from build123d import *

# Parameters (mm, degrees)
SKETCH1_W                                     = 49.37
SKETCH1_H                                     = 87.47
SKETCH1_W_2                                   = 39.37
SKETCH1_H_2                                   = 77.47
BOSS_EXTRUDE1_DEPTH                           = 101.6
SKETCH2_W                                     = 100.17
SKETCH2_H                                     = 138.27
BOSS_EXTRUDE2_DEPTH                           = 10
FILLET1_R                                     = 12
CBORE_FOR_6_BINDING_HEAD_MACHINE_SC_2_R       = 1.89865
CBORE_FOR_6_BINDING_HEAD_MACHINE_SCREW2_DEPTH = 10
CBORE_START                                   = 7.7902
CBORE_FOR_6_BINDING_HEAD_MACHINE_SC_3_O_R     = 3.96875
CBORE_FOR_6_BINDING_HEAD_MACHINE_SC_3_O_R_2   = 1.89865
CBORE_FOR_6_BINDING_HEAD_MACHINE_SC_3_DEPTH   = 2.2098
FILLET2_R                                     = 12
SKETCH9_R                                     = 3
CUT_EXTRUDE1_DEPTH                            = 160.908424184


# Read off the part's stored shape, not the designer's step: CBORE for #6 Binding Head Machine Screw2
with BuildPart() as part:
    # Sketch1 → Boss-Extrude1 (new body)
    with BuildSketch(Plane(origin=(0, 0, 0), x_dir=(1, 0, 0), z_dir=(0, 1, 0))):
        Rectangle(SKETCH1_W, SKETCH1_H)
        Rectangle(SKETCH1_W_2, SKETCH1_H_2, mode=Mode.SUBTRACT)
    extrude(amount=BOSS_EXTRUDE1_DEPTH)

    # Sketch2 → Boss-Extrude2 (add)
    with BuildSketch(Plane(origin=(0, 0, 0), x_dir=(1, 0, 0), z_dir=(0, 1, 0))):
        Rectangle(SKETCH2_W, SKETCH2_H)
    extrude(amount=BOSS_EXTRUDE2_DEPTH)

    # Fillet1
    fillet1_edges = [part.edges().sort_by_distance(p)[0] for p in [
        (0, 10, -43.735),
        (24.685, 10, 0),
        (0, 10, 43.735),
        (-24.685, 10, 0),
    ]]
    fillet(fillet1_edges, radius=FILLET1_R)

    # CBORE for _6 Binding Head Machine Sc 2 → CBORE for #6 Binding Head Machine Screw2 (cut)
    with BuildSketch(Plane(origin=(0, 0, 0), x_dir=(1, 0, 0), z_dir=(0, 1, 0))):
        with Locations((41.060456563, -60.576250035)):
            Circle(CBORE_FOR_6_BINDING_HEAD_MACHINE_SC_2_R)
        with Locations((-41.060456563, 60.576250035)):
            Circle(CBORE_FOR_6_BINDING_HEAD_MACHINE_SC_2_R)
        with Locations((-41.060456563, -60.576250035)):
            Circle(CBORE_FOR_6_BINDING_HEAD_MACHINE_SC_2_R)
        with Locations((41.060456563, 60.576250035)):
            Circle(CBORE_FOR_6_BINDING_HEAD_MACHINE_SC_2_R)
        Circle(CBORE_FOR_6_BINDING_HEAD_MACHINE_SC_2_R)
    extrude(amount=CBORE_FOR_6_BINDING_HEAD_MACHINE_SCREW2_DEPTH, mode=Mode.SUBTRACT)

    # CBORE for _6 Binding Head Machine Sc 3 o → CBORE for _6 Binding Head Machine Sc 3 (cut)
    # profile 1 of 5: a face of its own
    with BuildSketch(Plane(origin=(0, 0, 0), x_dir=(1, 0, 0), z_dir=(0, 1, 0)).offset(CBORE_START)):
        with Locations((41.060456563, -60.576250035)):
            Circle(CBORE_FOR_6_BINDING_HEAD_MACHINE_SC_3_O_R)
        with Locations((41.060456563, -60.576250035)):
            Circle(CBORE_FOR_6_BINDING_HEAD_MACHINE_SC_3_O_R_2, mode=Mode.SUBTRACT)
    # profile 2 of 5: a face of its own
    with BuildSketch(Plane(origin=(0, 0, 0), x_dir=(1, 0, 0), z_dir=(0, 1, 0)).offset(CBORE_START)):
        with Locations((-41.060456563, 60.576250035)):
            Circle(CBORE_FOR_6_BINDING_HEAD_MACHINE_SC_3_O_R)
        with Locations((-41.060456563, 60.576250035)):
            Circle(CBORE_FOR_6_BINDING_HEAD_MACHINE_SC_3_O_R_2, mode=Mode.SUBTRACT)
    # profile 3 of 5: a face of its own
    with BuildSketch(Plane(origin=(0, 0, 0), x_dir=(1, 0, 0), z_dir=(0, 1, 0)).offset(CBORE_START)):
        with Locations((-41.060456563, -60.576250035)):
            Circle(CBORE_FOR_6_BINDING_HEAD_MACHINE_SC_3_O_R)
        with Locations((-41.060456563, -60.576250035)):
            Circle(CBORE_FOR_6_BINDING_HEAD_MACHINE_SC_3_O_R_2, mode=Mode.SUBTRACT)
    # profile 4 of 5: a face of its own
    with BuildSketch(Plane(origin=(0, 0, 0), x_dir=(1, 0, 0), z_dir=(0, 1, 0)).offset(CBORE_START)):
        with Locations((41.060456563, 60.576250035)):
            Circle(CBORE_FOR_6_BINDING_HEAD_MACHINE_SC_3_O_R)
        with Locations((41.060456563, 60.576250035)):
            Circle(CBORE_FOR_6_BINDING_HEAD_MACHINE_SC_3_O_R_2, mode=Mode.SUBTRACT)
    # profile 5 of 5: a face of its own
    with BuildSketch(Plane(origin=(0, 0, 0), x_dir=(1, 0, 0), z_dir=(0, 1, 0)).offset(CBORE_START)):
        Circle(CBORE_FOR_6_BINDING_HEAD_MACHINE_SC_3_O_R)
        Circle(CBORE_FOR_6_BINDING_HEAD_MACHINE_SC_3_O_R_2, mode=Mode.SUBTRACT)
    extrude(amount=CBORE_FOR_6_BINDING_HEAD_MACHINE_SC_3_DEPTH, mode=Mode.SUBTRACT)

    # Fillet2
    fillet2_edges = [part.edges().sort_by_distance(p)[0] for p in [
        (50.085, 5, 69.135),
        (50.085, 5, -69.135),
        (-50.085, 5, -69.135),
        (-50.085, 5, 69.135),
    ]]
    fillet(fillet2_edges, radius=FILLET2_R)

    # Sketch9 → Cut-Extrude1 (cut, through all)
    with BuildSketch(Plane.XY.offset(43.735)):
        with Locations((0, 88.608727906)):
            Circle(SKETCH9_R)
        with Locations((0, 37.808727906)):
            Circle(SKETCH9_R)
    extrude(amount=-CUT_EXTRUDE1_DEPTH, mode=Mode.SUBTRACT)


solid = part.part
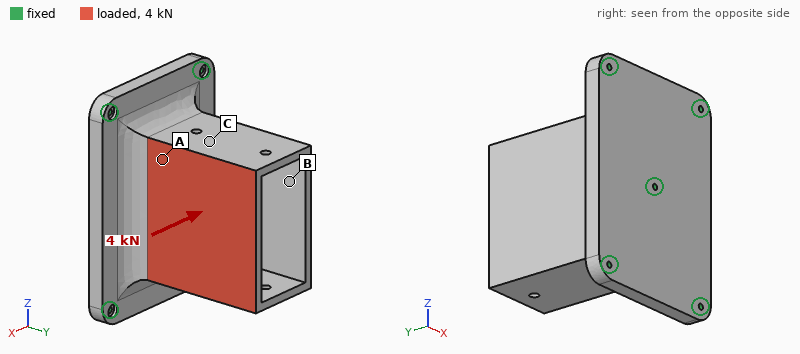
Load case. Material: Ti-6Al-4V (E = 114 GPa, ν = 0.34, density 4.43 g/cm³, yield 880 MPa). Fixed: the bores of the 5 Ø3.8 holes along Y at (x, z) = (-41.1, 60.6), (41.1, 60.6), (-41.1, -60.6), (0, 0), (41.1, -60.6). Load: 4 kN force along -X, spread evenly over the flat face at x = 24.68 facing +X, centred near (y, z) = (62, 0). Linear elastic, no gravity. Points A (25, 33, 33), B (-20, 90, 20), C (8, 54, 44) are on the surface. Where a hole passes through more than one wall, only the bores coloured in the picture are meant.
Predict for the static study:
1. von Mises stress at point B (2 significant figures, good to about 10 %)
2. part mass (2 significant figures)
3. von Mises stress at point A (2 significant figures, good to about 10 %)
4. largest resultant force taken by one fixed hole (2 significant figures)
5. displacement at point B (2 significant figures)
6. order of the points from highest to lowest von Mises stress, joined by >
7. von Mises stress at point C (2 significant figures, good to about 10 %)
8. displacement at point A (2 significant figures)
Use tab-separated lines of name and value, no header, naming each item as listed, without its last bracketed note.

von Mises stress at point B	9.2 MPa
part mass	1.2 kg
von Mises stress at point A	24 MPa
largest resultant force taken by one fixed hole	1.9 kN
displacement at point B	0.041 mm
order of the points from highest to lowest von Mises stress, joined by >	A > C > B
von Mises stress at point C	18 MPa
displacement at point A	0.026 mm
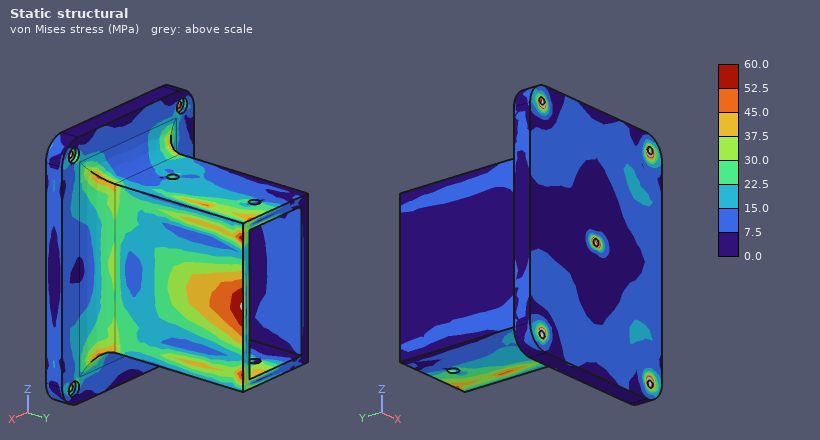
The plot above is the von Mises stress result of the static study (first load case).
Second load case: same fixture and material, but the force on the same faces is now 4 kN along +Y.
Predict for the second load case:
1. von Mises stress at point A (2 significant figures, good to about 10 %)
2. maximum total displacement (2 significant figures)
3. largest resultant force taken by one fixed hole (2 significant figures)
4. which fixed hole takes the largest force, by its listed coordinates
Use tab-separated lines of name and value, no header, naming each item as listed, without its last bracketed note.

von Mises stress at point A	9.6 MPa
maximum total displacement	41 µm
largest resultant force taken by one fixed hole	2.0 kN
which fixed hole takes the largest force, by its listed coordinates	(0, 0)
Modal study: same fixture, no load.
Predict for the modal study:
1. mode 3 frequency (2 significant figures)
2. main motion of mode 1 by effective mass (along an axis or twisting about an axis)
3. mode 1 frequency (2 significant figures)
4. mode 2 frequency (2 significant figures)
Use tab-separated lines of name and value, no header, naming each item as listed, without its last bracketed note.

mode 3 frequency	2900 Hz
main motion of mode 1 by effective mass	along X
mode 1 frequency	1900 Hz
mode 2 frequency	2800 Hz
